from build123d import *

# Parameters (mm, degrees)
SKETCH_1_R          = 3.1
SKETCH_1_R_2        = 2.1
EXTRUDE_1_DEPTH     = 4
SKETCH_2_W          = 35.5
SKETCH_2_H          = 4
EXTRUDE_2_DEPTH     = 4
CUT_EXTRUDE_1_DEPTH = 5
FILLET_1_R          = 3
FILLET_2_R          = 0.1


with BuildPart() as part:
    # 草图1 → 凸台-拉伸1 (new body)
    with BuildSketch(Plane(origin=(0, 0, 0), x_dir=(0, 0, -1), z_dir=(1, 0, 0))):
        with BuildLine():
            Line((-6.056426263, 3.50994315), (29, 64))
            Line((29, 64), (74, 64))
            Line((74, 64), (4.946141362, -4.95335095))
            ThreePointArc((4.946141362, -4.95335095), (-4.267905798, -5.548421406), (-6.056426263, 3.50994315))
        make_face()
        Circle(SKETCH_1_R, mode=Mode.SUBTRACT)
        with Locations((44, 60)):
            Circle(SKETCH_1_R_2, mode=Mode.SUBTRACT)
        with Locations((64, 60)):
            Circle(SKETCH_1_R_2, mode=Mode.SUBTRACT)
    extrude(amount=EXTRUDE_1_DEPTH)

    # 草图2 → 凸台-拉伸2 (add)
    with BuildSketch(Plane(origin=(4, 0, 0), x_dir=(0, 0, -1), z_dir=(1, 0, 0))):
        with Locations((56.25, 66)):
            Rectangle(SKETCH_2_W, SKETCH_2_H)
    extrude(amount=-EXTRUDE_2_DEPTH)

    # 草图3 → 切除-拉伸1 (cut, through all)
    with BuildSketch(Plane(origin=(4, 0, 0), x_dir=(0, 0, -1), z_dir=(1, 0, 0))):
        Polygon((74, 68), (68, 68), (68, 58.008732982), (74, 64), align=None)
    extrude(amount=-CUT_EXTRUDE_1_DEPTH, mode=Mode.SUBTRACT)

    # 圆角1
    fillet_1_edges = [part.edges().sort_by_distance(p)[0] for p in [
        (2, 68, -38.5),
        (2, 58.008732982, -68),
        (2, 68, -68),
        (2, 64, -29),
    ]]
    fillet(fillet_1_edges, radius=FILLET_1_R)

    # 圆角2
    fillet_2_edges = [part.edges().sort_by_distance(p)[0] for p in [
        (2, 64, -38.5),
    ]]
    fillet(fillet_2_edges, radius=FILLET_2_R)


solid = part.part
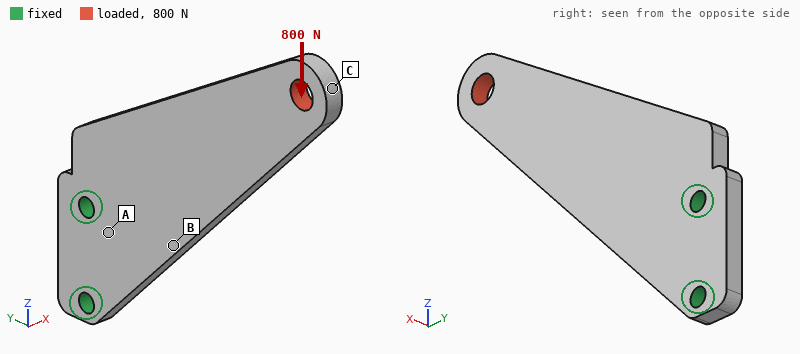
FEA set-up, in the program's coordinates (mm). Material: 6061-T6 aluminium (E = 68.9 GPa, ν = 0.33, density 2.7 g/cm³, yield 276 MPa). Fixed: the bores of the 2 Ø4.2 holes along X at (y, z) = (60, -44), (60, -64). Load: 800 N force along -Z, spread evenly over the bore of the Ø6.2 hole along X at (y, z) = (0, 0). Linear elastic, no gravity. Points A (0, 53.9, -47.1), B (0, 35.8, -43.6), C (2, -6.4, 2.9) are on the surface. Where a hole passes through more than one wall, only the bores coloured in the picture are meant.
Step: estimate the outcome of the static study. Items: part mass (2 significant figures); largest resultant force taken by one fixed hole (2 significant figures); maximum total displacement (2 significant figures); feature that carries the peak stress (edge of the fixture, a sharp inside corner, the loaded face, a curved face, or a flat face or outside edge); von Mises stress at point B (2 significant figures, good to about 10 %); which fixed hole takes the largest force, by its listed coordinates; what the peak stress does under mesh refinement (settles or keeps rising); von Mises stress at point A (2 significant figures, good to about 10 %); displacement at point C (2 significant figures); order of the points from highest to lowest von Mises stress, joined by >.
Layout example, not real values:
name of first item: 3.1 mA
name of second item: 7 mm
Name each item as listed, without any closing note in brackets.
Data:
part mass: 23 g
largest resultant force taken by one fixed hole: 2.4 kN
maximum total displacement: 0.36 mm
feature that carries the peak stress: a sharp inside corner
von Mises stress at point B: 69 MPa
which fixed hole takes the largest force, by its listed coordinates: (60, -64)
what the peak stress does under mesh refinement: keeps rising
von Mises stress at point A: 32 MPa
displacement at point C: 0.36 mm
order of the points from highest to lowest von Mises stress, joined by >: B > A > C
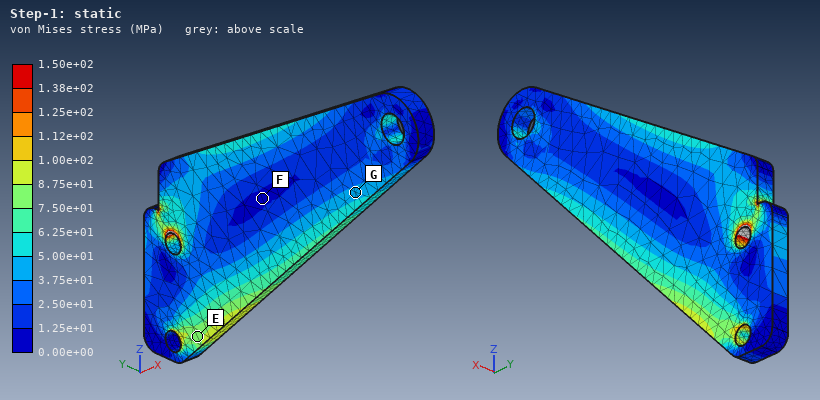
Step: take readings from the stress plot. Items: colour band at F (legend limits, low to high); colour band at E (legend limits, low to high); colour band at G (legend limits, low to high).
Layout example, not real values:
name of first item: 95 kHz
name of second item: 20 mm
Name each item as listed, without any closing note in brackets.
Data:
colour band at F: 0.00e+00 to 1.25e+01 MPa
colour band at E: 7.50e+01 to 8.75e+01 MPa
colour band at G: 3.75e+01 to 5.00e+01 MPa
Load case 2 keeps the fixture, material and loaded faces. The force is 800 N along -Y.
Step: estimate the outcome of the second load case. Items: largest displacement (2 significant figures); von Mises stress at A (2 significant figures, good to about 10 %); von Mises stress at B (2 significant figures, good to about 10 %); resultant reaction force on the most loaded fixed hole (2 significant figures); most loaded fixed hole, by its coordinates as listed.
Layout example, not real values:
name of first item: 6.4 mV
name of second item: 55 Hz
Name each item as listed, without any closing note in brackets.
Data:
largest displacement: 0.28 mm
von Mises stress at A: 23 MPa
von Mises stress at B: 45 MPa
resultant reaction force on the most loaded fixed hole: 2.4 kN
most loaded fixed hole, by its coordinates as listed: (60, -44)
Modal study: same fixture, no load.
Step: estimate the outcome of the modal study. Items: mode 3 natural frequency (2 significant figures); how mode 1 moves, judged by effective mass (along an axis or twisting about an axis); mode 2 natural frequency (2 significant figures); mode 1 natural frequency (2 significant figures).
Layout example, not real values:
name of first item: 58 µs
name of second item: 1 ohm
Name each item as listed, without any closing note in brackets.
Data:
mode 3 natural frequency: 3400 Hz
how mode 1 moves, judged by effective mass: along X
mode 2 natural frequency: 3400 Hz
mode 1 natural frequency: 670 Hz
